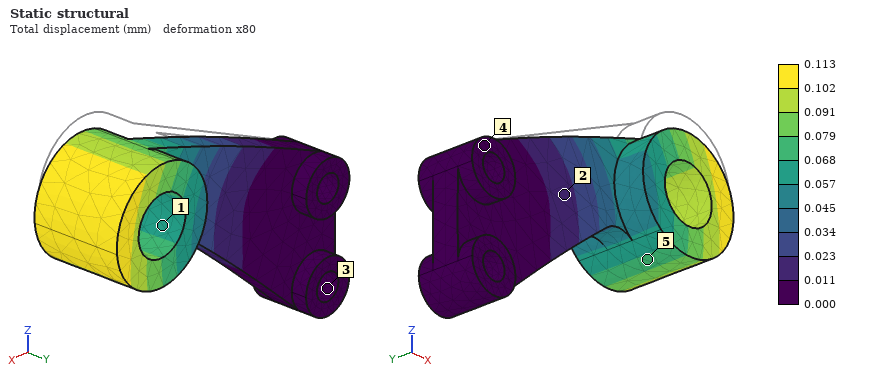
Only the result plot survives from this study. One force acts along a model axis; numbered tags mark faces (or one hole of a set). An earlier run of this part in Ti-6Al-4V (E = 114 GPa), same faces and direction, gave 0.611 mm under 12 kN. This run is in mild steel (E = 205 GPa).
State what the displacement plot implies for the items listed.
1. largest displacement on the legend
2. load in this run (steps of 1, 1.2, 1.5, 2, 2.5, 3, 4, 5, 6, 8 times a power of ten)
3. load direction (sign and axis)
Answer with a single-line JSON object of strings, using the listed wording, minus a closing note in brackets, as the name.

{"largest displacement on the legend": "0.113 mm", "load in this run": "4 kN", "load direction": "-Z"}
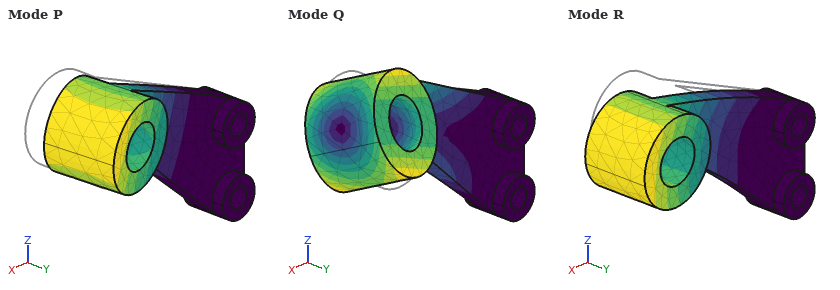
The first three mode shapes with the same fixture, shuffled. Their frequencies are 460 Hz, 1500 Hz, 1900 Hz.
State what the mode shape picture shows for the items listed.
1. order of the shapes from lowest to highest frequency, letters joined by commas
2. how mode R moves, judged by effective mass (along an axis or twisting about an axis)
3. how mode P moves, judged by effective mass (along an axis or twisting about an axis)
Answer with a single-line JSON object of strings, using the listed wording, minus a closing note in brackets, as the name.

{"order of the shapes from lowest to highest frequency, letters joined by commas": "P, R, Q", "how mode R moves, judged by effective mass": "along Z", "how mode P moves, judged by effective mass": "along Y"}
